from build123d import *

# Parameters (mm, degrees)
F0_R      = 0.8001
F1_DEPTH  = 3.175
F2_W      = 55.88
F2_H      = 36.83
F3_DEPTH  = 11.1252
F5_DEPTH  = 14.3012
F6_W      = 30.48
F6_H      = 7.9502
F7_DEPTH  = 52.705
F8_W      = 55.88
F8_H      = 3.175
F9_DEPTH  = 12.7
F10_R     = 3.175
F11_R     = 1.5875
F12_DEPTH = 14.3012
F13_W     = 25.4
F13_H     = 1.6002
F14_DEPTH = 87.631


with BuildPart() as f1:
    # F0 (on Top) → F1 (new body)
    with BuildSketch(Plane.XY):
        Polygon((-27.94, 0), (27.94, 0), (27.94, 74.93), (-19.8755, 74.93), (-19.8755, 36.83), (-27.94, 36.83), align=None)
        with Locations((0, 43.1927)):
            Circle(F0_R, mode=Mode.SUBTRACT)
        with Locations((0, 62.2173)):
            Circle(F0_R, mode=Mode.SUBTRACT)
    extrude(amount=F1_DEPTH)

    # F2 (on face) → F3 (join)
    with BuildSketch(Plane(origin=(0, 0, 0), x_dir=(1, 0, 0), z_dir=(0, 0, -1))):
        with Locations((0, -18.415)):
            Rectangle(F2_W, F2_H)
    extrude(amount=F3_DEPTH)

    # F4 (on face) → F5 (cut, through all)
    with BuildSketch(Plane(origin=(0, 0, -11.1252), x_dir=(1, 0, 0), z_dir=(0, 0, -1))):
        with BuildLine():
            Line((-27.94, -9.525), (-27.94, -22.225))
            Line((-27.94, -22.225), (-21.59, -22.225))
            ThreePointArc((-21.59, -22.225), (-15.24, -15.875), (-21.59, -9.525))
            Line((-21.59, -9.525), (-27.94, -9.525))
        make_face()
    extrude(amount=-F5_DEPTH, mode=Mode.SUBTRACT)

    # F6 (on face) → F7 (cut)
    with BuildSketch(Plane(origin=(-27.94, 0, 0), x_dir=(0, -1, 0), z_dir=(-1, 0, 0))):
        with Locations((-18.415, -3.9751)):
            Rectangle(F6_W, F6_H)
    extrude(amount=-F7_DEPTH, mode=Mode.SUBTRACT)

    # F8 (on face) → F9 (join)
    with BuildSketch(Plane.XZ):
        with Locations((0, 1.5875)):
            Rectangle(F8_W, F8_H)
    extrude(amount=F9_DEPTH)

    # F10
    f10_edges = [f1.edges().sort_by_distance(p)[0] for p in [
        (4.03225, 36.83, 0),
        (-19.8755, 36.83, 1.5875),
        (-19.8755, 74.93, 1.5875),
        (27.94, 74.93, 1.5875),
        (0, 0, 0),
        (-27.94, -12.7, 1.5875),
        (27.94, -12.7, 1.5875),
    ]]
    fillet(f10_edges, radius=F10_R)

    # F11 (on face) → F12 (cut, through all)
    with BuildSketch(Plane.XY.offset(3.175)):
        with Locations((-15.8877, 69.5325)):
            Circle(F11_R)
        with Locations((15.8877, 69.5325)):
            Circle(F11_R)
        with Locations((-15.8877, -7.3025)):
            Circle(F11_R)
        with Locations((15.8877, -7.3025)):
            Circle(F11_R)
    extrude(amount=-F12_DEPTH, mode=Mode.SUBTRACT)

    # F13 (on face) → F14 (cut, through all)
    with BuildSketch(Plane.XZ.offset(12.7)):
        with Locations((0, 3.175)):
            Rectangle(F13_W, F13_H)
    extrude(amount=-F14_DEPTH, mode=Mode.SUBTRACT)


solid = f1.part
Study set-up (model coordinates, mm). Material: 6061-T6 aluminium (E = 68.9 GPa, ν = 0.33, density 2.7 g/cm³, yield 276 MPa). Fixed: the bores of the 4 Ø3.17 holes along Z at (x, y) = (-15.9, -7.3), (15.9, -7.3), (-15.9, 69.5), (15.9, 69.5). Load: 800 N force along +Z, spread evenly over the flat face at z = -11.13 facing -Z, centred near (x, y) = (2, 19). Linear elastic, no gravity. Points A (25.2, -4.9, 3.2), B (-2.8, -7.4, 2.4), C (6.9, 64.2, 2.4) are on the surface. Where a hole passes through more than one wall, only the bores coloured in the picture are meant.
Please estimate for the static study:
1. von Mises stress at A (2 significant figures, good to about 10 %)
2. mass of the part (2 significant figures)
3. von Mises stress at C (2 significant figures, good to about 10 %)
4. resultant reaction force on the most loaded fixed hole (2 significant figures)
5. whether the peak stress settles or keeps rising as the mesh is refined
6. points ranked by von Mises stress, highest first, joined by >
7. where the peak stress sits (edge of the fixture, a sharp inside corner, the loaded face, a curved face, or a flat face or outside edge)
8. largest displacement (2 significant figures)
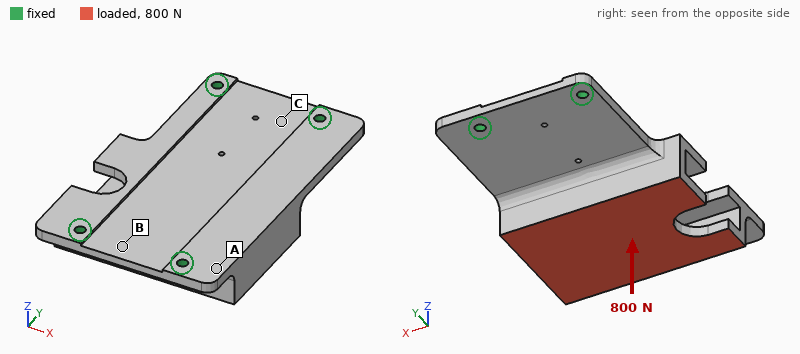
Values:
15 MPa
60 g
25 MPa
310 N
keeps rising
C > A > B
edge of the fixture
0.12 mm
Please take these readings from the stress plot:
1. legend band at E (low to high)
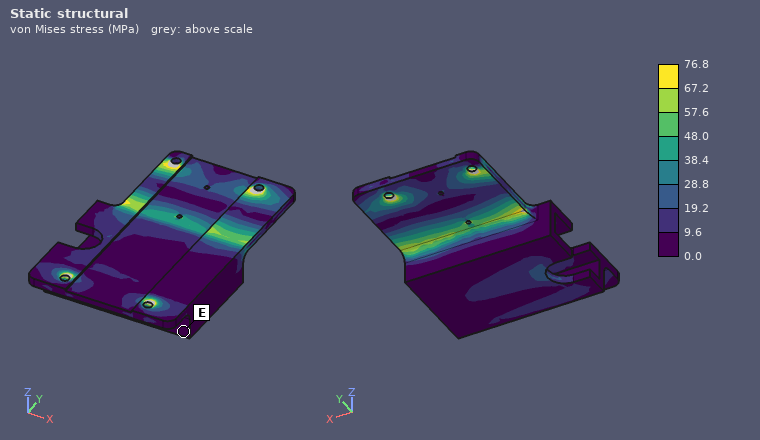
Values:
0.0 to 9.6 MPa
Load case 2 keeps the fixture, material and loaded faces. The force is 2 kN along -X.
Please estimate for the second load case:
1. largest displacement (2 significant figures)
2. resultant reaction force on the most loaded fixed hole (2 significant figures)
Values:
90 µm
1.3 kN
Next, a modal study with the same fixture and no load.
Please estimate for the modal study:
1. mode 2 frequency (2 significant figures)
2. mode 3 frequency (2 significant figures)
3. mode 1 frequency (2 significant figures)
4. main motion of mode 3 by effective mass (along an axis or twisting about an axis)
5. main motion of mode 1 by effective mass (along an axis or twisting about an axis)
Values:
4400 Hz
8200 Hz
2100 Hz
along Y
along Z
